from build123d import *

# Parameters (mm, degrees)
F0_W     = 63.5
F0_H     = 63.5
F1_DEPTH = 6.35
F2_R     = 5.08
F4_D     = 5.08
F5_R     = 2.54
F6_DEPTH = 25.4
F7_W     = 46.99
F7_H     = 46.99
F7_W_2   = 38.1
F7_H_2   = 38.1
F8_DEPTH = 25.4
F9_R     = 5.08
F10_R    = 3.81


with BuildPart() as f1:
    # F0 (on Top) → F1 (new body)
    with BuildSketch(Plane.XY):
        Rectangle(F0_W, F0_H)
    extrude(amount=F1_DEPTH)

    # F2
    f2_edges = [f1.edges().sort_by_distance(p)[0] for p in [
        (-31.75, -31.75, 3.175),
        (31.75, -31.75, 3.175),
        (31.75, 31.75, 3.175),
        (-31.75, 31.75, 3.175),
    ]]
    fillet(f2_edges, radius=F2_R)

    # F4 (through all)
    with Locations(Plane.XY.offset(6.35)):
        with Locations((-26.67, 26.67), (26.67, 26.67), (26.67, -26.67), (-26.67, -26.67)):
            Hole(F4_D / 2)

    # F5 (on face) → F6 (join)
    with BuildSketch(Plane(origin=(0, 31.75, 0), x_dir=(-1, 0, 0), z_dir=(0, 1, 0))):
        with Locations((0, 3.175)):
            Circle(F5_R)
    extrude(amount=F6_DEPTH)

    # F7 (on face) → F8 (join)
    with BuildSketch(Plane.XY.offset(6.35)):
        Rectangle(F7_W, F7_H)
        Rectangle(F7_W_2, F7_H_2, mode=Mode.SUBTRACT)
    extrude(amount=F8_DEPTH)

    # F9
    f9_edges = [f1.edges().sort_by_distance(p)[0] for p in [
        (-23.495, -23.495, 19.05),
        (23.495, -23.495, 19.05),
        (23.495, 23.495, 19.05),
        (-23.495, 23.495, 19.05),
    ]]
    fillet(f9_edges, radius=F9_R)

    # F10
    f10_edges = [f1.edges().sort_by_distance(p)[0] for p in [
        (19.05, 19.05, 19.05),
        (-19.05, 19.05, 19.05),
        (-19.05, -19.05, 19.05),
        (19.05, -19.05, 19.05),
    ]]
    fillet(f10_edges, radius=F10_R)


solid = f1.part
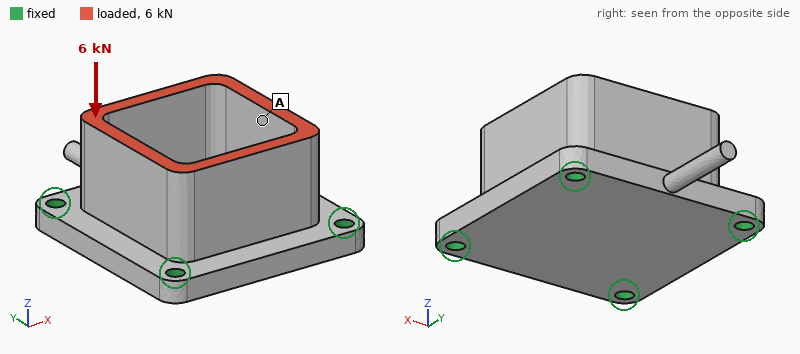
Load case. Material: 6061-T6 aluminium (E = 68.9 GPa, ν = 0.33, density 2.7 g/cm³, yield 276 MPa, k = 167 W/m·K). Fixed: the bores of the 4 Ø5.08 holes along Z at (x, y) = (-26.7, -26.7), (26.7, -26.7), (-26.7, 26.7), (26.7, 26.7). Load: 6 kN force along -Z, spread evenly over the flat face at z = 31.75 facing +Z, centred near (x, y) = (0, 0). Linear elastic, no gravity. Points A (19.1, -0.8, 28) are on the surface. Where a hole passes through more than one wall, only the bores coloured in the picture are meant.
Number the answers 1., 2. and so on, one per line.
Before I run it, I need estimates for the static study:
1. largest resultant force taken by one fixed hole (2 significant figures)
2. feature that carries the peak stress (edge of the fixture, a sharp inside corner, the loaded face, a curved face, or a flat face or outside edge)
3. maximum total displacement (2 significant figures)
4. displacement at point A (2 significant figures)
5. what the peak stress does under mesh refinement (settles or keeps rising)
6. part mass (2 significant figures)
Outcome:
1. 1.6 kN
2. edge of the fixture
3. 19 µm
4. 16 µm
5. keeps rising
6. 120 g
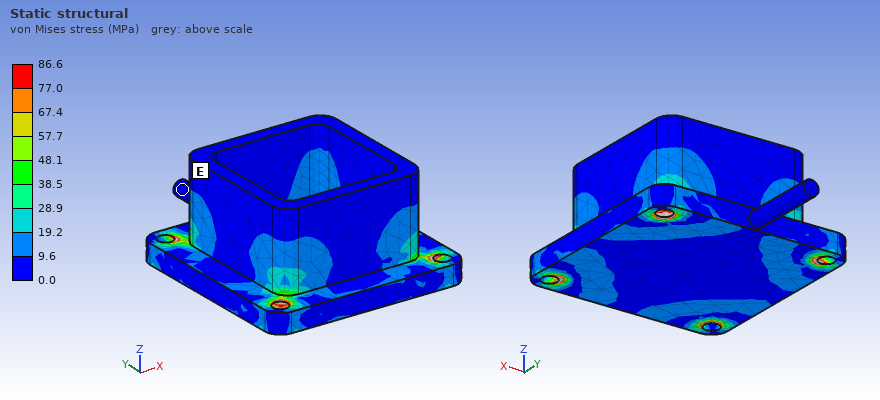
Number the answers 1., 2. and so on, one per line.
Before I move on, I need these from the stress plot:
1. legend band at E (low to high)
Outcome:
1. 0.0 to 9.6 MPa
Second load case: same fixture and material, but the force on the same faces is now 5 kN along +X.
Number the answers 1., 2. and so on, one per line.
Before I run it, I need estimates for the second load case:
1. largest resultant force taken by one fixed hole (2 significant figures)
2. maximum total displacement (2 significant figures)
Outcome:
1. 2.0 kN
2. 97 µm
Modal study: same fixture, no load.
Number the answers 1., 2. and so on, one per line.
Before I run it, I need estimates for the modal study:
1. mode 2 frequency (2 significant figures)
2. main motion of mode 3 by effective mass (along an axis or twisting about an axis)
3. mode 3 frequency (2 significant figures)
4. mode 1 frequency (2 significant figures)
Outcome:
1. 5000 Hz
2. along Z
3. 9300 Hz
4. 4500 Hz
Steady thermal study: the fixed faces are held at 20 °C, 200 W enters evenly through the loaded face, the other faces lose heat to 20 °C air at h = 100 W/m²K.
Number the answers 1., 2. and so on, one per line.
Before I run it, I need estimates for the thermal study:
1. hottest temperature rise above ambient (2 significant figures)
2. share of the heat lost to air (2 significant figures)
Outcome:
1. 59 K
2. 24 %
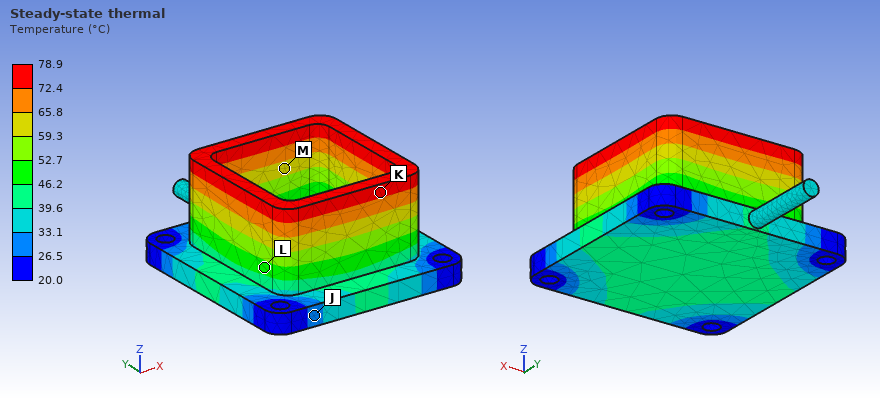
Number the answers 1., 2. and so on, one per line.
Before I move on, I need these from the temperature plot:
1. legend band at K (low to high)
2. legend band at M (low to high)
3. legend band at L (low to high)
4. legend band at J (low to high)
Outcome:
1. 72.4 to 78.9 °C
2. 59.3 to 65.8 °C
3. 46.2 to 52.7 °C
4. 26.5 to 33.1 °C
